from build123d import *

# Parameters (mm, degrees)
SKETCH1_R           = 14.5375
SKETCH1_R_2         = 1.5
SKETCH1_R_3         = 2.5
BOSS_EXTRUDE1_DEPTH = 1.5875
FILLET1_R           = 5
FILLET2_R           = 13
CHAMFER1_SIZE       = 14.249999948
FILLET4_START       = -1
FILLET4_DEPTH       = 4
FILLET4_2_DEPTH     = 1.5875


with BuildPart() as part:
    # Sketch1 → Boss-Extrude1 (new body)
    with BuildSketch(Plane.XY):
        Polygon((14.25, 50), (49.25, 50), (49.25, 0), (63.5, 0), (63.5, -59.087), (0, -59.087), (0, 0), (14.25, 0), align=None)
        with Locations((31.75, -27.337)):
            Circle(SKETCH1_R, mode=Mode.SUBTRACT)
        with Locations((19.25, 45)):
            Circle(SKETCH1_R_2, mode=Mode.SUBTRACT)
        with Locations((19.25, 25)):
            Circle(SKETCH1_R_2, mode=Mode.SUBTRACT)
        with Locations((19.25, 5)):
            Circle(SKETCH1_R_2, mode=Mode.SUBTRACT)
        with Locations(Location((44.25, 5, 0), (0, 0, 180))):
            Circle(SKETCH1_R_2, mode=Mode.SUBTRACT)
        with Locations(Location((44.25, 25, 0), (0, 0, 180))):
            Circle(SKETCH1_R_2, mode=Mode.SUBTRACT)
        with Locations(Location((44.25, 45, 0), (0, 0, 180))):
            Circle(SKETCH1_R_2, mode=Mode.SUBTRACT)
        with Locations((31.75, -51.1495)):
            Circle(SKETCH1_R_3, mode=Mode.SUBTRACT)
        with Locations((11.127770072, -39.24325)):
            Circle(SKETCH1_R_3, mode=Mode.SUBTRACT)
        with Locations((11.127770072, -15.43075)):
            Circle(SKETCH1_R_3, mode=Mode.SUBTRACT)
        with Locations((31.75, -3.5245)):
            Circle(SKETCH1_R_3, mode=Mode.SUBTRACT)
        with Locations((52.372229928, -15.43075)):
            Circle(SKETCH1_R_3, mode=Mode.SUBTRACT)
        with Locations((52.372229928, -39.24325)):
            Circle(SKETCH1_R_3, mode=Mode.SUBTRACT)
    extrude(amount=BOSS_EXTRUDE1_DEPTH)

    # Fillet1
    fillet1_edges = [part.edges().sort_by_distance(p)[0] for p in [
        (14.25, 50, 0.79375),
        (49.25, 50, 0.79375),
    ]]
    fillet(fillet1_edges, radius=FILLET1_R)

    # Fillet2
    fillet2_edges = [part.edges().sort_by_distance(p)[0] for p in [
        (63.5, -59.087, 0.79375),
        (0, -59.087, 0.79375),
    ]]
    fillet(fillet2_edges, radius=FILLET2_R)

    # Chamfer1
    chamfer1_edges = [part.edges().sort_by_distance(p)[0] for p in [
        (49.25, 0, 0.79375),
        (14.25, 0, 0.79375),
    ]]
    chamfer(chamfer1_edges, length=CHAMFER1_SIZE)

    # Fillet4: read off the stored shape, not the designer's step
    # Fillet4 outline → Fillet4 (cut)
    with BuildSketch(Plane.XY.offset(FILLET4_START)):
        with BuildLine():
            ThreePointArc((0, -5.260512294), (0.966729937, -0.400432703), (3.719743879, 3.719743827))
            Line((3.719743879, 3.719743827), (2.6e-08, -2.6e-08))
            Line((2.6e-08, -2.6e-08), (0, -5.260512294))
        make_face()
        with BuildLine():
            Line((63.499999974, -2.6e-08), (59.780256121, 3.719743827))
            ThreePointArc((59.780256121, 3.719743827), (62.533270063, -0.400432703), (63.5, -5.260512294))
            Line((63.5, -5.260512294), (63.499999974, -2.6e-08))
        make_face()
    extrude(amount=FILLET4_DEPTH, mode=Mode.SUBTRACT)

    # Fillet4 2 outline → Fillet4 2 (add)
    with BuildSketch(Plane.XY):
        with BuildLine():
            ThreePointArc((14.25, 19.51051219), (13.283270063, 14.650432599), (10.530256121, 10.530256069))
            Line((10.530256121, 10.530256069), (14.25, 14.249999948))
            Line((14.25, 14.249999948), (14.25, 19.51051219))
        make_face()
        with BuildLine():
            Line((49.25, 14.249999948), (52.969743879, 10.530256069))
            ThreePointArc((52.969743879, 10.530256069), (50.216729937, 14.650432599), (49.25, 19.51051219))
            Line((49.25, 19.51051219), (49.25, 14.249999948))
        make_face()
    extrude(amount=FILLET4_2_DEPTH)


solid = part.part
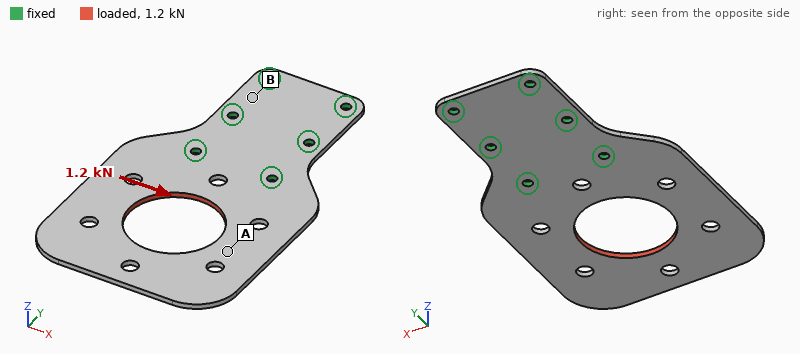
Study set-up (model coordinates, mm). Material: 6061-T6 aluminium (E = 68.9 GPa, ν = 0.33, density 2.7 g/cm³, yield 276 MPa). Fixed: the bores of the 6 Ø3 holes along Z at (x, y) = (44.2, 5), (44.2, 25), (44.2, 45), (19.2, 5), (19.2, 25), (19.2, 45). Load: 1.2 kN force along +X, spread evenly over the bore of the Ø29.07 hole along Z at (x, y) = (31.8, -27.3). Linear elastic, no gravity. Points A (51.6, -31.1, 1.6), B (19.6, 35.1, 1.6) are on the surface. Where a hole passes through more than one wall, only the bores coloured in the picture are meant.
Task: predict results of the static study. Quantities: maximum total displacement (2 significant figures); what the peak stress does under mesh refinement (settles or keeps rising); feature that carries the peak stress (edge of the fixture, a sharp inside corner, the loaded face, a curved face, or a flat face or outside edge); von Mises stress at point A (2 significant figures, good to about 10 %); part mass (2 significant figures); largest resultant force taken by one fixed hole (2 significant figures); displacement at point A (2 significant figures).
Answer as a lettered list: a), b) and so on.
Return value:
a) 0.14 mm
b) keeps rising
c) edge of the fixture
d) 23 MPa
e) 21 g
f) 1.2 kN
g) 0.092 mm
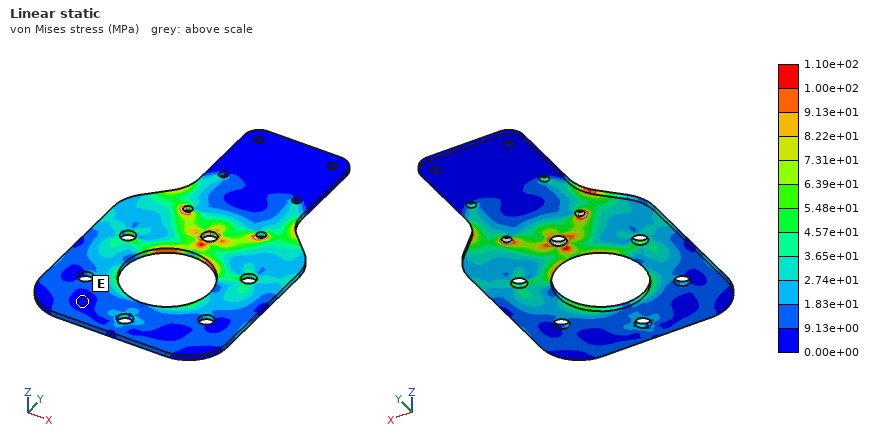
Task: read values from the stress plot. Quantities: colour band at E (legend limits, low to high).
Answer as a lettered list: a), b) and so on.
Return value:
a) 0.00e+00 to 9.13e+00 MPa
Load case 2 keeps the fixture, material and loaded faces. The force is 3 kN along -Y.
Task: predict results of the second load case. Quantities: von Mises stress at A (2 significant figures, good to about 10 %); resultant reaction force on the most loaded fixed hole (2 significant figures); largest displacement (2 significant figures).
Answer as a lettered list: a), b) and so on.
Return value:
a) 26 MPa
b) 1.2 kN
c) 57 µm
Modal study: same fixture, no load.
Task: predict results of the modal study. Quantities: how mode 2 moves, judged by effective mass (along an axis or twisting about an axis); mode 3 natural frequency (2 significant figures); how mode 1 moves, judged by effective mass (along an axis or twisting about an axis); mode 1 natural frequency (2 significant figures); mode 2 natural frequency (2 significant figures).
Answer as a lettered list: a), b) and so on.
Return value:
a) twisting about Y
b) 1600 Hz
c) along Z
d) 290 Hz
e) 660 Hz
